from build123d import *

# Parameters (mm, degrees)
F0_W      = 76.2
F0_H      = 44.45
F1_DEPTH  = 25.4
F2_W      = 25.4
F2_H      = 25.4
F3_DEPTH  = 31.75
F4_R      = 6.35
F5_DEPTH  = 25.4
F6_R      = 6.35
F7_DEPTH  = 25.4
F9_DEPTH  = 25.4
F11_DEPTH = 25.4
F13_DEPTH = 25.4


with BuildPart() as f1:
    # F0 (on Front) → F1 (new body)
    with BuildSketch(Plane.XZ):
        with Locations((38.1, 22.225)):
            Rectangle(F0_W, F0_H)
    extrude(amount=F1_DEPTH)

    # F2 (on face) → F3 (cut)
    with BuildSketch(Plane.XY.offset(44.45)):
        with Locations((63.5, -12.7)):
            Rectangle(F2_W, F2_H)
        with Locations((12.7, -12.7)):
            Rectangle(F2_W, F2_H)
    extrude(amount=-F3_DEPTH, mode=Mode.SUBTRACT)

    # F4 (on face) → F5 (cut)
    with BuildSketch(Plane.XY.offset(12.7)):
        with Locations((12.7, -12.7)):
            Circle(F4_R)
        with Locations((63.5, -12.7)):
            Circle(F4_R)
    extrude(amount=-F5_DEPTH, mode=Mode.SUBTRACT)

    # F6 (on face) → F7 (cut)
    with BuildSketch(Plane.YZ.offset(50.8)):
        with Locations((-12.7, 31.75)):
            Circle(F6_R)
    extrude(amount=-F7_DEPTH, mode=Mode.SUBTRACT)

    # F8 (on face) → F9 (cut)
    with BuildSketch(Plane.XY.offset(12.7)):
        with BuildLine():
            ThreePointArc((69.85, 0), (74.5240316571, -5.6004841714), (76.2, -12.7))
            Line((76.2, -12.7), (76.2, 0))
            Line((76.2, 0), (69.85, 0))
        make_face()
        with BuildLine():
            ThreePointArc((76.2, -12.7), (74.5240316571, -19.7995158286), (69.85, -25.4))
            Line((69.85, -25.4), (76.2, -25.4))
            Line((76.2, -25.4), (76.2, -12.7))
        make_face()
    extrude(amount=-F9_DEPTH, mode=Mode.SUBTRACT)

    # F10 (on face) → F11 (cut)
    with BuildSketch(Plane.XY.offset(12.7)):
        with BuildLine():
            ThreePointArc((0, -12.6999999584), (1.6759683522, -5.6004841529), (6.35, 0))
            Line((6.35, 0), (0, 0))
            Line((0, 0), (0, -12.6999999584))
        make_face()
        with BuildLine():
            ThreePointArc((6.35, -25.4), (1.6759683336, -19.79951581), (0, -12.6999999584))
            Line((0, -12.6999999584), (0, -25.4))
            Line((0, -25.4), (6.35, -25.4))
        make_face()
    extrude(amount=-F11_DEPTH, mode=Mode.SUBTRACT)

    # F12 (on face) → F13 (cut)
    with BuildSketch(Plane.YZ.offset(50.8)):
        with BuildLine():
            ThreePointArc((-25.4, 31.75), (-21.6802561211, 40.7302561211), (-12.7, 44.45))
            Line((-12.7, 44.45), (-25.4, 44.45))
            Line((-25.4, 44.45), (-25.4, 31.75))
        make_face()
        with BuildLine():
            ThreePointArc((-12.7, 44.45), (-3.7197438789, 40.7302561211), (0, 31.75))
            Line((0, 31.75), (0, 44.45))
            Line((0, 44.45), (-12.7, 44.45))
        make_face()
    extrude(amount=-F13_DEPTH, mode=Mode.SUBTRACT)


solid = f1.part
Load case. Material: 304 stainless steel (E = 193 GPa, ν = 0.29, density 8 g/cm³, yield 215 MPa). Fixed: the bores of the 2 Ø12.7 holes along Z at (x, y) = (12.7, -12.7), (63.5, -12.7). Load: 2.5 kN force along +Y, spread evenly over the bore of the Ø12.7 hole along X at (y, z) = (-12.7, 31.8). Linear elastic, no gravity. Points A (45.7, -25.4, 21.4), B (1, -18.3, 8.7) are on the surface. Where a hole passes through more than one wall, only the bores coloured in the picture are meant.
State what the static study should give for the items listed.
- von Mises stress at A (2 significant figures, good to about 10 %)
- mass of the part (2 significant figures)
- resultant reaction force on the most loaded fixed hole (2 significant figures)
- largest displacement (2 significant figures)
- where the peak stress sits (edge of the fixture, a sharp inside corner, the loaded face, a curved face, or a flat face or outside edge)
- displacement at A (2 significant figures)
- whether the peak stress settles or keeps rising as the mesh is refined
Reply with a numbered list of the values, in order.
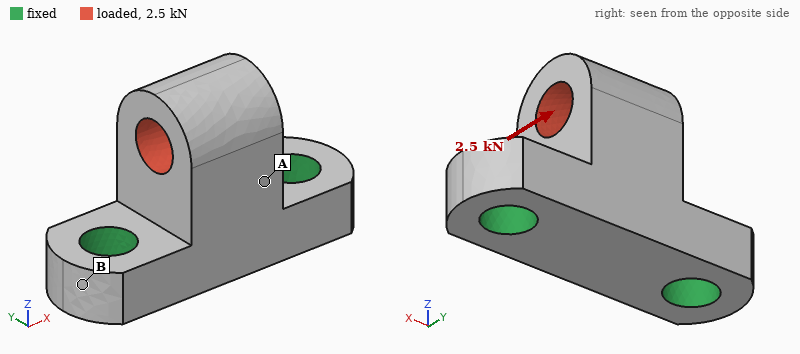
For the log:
1. 15 MPa
2. 290 g
3. 1.3 kN
4. 19 µm
5. edge of the fixture
6. 9.1 µm
7. keeps rising
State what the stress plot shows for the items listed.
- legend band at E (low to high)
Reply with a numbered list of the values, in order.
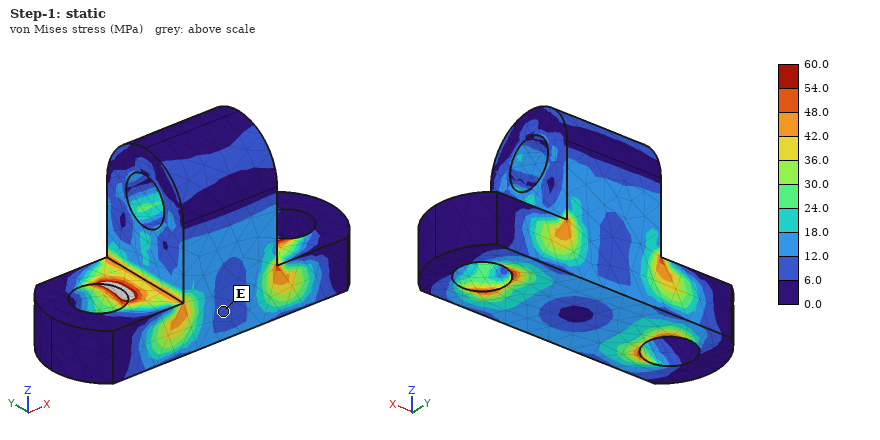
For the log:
1. 6.0 to 12.0 MPa
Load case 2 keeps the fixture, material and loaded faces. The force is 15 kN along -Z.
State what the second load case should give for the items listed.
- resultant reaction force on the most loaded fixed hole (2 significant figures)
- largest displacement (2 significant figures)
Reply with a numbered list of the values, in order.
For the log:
1. 7.8 kN
2. 12 µm
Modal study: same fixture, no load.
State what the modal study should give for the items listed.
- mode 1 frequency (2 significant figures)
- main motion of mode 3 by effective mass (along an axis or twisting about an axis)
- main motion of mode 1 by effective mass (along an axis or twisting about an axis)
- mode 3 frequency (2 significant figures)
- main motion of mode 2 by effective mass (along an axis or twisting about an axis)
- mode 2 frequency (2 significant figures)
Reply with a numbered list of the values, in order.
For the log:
1. 6800 Hz
2. along Z
3. along Y
4. 17 kHz
5. along X
6. 12 kHz
